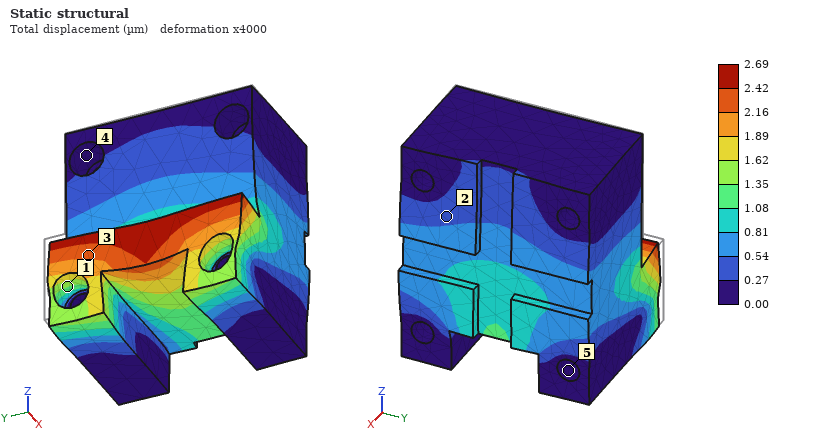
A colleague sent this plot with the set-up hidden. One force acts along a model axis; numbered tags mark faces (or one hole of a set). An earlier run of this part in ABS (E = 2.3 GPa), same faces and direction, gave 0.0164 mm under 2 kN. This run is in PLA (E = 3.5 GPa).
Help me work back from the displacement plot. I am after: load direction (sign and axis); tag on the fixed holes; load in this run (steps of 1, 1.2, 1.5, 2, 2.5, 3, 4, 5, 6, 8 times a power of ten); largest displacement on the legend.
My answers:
+X
5
500 N
2.69 µm
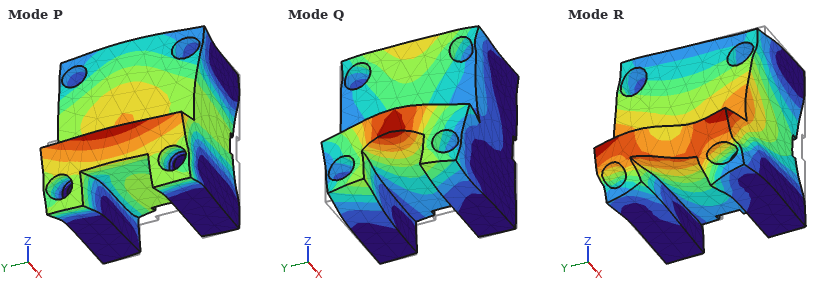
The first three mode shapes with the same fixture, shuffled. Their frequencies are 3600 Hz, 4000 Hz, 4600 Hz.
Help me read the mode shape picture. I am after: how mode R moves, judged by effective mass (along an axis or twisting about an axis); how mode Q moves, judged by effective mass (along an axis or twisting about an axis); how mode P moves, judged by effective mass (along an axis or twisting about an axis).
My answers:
along Y
along Z
along X
